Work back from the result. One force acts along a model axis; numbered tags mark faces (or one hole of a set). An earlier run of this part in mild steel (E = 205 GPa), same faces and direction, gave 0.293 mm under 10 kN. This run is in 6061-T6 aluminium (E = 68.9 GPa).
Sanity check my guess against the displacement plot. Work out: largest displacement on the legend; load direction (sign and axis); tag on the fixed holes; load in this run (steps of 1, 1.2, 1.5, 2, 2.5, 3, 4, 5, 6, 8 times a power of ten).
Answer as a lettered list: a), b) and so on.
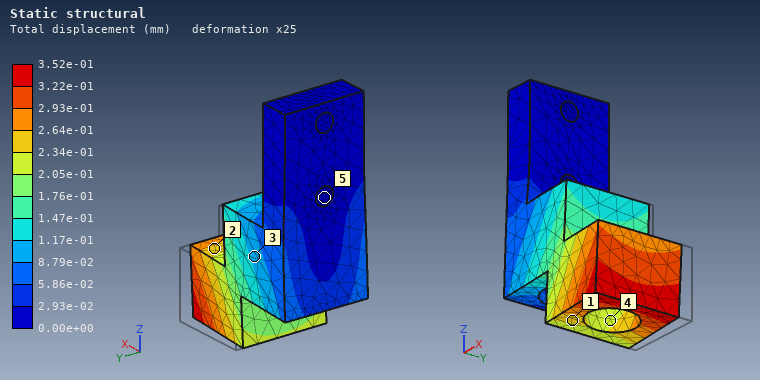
a) 3.52e-01 mm
b) -Y
c) 5
d) 4 kN
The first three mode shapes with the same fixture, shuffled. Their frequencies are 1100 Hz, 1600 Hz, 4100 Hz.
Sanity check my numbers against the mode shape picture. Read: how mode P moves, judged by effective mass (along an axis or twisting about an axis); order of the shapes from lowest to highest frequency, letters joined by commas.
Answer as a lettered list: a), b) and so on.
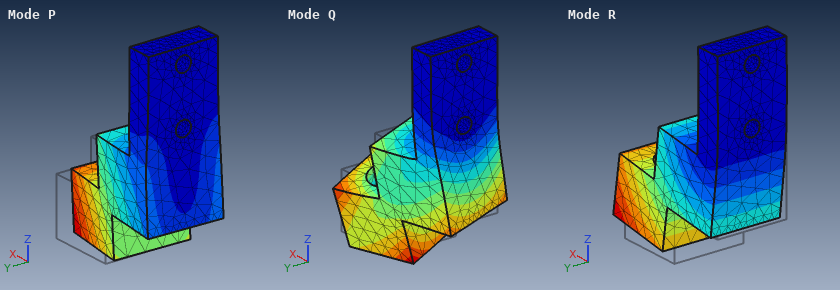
a) along Y
b) R, P, Q
